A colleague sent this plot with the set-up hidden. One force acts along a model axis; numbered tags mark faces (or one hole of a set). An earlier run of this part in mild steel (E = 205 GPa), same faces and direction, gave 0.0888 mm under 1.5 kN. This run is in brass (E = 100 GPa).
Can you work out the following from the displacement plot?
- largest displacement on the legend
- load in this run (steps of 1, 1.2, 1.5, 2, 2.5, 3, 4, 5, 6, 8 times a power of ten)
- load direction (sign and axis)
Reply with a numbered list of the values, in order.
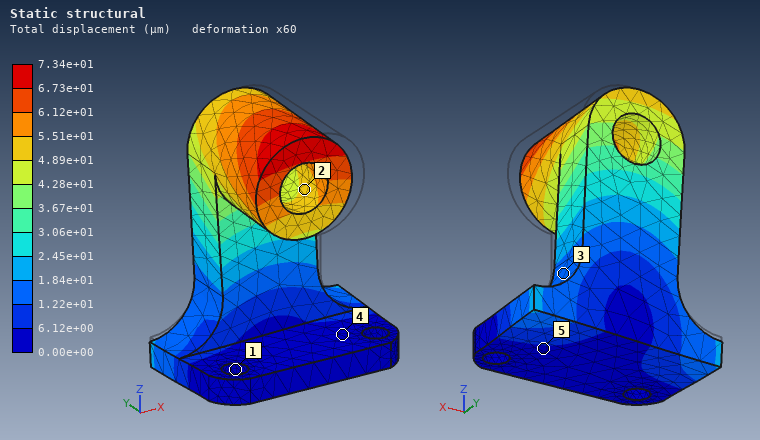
1. 7.34e+01 µm
2. 600 N
3. -X
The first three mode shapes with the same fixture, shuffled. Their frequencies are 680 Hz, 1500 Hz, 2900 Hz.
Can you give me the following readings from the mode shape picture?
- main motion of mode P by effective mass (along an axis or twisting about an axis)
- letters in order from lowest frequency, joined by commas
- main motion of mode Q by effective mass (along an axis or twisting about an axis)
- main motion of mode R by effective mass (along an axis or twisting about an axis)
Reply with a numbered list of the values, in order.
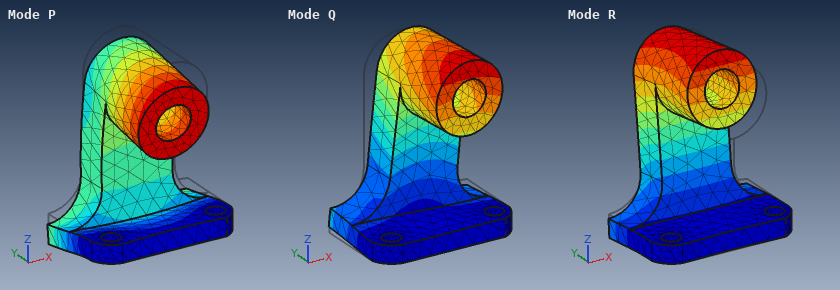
1. along Z
2. R, Q, P
3. along X
4. along Y
